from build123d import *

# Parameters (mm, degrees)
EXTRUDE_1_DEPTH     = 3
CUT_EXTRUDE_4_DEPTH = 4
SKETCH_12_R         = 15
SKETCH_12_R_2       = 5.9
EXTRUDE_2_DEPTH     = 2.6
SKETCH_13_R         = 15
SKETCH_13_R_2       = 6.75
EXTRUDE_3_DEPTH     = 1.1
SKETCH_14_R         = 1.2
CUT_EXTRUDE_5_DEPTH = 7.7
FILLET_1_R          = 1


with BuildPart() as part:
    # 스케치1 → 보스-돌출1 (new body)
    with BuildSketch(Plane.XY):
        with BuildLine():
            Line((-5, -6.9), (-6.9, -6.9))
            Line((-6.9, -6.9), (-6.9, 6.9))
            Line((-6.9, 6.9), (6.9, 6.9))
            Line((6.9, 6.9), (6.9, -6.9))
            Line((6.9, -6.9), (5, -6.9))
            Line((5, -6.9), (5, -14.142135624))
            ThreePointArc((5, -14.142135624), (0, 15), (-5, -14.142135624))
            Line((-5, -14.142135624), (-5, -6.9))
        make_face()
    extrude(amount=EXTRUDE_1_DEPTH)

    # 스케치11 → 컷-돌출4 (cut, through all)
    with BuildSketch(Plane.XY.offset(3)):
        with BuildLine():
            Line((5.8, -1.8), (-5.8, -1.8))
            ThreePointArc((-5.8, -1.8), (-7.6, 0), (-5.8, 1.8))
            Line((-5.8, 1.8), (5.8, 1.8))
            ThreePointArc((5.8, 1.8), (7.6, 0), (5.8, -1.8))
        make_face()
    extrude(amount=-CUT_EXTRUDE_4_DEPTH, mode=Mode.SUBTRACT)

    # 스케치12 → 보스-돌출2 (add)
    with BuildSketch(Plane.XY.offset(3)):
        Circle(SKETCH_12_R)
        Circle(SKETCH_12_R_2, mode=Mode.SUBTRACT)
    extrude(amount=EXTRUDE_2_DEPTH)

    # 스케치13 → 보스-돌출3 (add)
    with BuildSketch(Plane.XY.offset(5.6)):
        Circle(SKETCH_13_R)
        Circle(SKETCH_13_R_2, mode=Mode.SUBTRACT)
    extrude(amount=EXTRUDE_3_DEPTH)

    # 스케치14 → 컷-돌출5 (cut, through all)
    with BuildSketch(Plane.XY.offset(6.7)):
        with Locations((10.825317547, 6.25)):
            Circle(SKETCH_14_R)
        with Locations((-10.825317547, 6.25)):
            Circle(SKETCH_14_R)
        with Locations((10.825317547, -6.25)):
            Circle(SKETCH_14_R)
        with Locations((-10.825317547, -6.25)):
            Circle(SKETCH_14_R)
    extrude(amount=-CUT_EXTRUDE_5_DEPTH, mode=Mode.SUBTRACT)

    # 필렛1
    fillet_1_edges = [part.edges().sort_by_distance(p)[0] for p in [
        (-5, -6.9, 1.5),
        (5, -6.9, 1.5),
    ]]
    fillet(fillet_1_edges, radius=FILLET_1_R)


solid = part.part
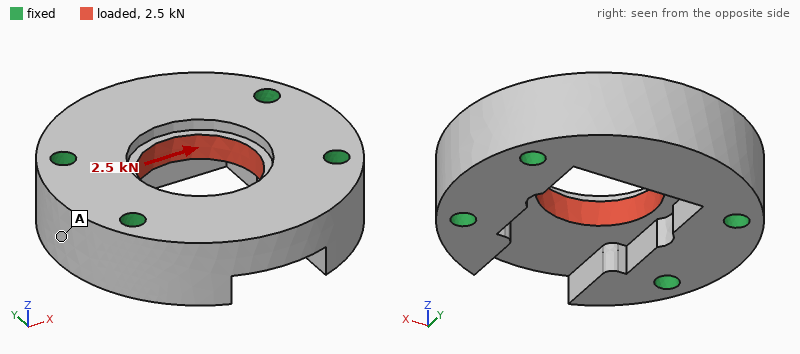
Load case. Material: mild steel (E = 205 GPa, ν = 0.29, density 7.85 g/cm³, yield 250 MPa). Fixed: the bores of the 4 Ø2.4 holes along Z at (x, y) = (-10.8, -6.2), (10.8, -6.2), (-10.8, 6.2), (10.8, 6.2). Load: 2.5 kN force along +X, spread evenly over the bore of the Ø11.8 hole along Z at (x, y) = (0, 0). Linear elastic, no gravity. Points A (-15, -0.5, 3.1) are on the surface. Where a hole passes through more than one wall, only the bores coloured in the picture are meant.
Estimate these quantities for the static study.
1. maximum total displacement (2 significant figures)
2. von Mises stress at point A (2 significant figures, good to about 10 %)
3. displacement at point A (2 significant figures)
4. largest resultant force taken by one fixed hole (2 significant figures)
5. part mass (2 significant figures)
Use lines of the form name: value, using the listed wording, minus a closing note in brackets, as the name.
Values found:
maximum total displacement: 1.0 µm
von Mises stress at point A: 7.1 MPa
displacement at point A: 0.28 µm
largest resultant force taken by one fixed hole: 640 N
part mass: 26 g
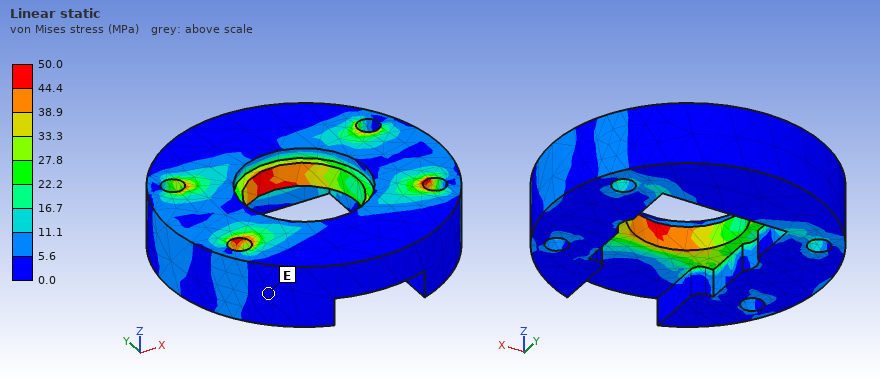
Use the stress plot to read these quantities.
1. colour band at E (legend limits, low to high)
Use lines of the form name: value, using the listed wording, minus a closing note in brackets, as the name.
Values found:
colour band at E: 0.0 to 5.6 MPa
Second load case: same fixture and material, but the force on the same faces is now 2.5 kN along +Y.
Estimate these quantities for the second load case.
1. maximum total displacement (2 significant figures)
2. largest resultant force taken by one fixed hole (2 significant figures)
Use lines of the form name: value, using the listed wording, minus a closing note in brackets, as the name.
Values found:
maximum total displacement: 1.9 µm
largest resultant force taken by one fixed hole: 640 N
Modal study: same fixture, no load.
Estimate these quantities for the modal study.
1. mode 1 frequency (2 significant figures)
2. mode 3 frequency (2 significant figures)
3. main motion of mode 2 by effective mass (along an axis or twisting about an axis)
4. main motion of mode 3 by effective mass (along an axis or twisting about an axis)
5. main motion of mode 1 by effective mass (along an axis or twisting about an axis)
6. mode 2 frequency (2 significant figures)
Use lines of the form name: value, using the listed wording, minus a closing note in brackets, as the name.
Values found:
mode 1 frequency: 37 kHz
mode 3 frequency: 62 kHz
main motion of mode 2 by effective mass: along Z
main motion of mode 3 by effective mass: along Y
main motion of mode 1 by effective mass: along Z
mode 2 frequency: 41 kHz
